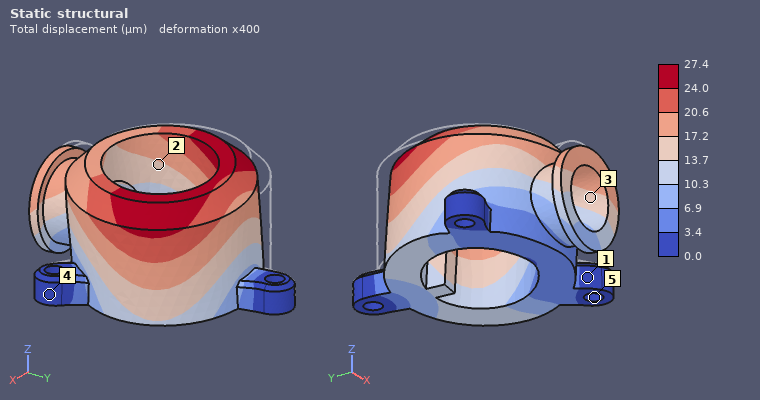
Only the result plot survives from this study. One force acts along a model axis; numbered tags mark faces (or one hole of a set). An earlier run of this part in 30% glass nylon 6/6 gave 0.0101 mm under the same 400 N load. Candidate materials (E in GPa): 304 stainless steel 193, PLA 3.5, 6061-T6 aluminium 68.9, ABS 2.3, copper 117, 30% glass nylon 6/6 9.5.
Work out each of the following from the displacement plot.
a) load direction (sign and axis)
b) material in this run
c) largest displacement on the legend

+X
PLA
27.4 µm
